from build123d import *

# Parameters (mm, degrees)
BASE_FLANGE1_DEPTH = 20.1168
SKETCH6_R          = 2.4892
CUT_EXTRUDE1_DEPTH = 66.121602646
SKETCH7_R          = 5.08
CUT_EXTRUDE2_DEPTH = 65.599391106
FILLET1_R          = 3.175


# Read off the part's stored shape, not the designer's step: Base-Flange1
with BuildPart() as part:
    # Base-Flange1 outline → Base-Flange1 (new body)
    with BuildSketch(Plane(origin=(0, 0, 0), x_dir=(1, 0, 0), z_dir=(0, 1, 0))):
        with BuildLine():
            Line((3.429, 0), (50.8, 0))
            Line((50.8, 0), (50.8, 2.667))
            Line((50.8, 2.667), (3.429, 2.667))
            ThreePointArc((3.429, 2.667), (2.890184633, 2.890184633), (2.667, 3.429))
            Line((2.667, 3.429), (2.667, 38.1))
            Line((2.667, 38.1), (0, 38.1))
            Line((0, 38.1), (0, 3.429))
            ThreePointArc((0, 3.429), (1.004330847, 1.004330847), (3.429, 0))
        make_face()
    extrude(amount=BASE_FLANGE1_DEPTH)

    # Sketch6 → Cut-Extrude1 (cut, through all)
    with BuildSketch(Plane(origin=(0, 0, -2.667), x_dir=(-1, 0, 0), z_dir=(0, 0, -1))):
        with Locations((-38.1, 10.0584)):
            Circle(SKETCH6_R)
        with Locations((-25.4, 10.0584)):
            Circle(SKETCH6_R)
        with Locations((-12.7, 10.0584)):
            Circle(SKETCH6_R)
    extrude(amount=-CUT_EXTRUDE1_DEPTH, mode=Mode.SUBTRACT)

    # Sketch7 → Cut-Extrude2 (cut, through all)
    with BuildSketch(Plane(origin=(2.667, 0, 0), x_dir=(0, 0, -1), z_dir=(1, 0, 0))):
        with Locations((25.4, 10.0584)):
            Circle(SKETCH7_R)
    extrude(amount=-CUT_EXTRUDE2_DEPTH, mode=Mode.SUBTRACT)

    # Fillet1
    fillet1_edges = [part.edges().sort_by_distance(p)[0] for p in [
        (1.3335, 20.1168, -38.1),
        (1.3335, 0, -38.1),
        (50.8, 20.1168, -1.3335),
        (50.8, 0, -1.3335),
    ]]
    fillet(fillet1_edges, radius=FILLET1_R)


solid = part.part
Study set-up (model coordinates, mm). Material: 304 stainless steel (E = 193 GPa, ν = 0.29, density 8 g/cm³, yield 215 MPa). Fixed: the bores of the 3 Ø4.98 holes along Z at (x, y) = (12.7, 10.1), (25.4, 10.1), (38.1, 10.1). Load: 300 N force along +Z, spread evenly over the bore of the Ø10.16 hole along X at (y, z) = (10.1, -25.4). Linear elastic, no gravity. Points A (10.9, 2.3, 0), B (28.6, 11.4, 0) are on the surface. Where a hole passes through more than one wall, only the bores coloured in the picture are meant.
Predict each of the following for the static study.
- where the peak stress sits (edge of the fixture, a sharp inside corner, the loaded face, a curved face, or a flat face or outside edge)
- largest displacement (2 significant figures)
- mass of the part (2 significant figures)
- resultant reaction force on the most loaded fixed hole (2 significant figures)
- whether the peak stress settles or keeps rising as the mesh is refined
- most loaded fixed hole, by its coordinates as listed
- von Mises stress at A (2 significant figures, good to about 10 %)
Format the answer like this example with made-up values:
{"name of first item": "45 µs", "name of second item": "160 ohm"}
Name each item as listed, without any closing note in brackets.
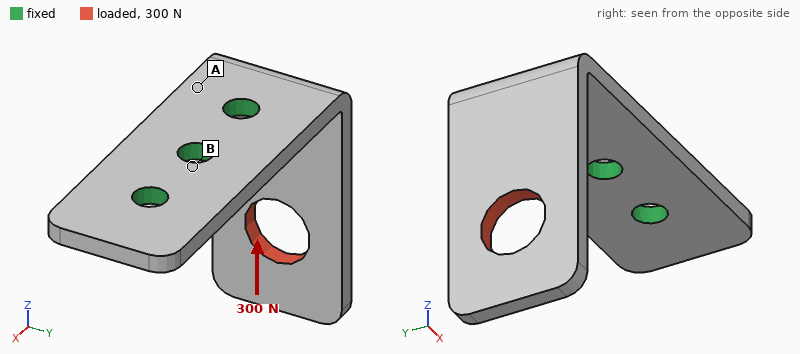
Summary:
{"where the peak stress sits": "edge of the fixture", "largest displacement": "99 µm", "mass of the part": "33 g", "resultant reaction force on the most loaded fixed hole": "350 N", "whether the peak stress settles or keeps rising as the mesh is refined": "keeps rising", "most loaded fixed hole, by its coordinates as listed": "(12.7, 10.1)", "von Mises stress at A": "57 MPa"}
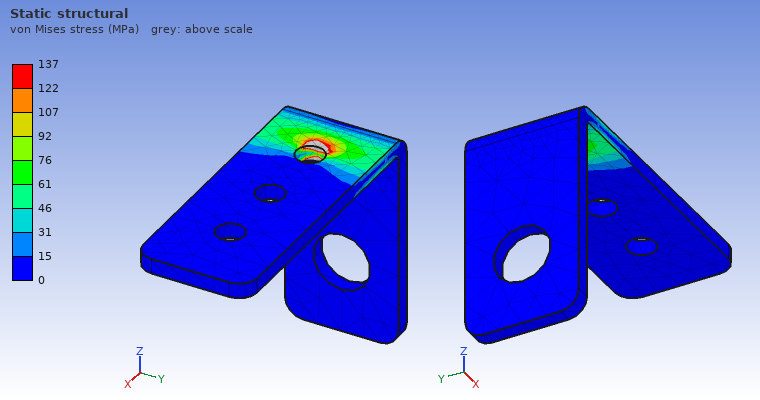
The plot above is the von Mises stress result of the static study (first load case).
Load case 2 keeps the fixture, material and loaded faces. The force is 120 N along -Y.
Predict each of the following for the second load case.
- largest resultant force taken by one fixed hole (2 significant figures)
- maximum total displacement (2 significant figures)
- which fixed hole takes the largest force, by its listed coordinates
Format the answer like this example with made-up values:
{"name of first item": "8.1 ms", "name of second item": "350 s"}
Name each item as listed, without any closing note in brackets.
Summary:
{"largest resultant force taken by one fixed hole": "170 N", "maximum total displacement": "97 µm", "which fixed hole takes the largest force, by its listed coordinates": "(12.7, 10.1)"}
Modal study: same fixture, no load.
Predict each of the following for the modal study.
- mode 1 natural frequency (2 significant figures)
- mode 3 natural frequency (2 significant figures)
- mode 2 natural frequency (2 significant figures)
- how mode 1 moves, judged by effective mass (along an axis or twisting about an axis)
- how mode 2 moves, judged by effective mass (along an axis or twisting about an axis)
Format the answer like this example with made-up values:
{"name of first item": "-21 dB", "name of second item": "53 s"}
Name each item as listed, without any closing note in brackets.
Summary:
{"mode 1 natural frequency": "1200 Hz", "mode 3 natural frequency": "5500 Hz", "mode 2 natural frequency": "2100 Hz", "how mode 1 moves, judged by effective mass": "along X", "how mode 2 moves, judged by effective mass": "along Y"}
